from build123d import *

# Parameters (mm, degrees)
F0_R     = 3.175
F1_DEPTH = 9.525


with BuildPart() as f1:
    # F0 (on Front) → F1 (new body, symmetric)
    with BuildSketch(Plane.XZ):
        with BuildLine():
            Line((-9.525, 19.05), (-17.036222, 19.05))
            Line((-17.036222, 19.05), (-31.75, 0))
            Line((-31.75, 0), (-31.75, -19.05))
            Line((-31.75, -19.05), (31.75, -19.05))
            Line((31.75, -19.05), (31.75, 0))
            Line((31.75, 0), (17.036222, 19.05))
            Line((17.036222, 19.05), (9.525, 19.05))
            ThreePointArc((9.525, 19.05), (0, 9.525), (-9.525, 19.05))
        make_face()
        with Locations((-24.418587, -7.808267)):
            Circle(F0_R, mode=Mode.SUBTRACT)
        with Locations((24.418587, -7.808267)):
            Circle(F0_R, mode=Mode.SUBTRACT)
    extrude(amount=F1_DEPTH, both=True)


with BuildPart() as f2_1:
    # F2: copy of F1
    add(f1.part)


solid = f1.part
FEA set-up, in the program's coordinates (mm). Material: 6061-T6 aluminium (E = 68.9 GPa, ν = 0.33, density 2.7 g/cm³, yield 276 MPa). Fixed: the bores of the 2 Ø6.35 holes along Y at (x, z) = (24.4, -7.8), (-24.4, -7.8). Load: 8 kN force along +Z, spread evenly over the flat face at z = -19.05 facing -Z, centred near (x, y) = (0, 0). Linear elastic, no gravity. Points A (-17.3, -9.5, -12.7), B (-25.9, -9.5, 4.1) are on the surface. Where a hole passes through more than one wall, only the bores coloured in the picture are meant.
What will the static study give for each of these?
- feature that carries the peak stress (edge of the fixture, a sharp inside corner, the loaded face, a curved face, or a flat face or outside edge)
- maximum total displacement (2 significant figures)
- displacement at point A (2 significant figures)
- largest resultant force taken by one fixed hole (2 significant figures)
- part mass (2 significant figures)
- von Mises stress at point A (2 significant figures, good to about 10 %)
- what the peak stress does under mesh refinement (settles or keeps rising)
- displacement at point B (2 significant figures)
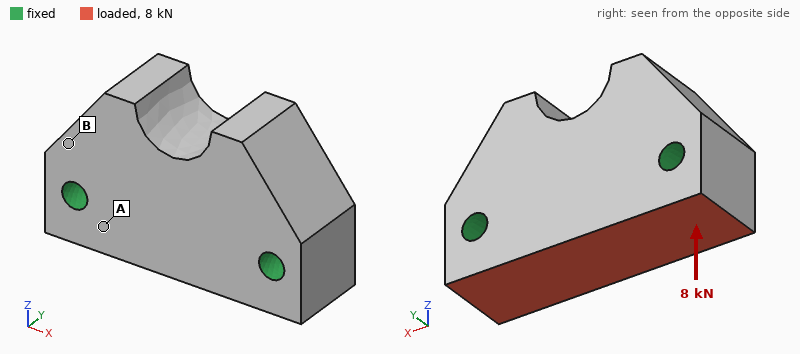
edge of the fixture
5.5 µm
2.3 µm
4.0 kN
99 g
10 MPa
keeps rising
0.96 µm
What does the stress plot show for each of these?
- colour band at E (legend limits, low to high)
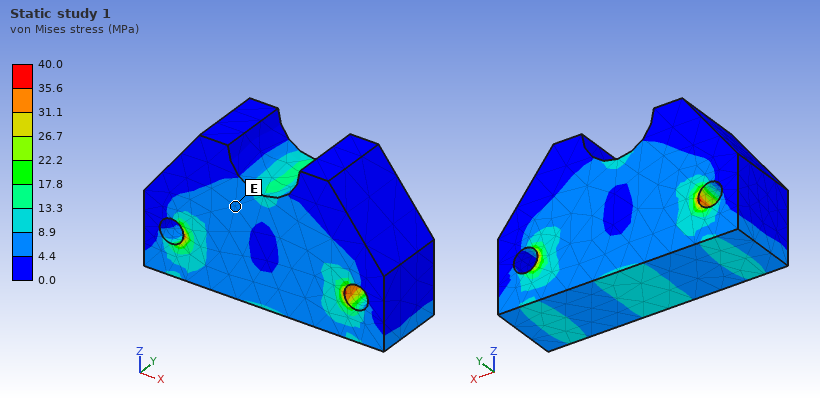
4.4 to 8.9 MPa
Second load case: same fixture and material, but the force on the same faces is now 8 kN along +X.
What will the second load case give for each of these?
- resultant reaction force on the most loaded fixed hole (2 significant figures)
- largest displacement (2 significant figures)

4.3 kN
5.9 µm
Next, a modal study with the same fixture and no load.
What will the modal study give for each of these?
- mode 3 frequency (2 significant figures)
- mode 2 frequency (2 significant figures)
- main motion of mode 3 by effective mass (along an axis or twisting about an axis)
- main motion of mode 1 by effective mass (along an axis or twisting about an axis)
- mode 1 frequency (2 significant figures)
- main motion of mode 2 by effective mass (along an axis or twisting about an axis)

24 kHz
21 kHz
along Y
along Y
16 kHz
along Z
